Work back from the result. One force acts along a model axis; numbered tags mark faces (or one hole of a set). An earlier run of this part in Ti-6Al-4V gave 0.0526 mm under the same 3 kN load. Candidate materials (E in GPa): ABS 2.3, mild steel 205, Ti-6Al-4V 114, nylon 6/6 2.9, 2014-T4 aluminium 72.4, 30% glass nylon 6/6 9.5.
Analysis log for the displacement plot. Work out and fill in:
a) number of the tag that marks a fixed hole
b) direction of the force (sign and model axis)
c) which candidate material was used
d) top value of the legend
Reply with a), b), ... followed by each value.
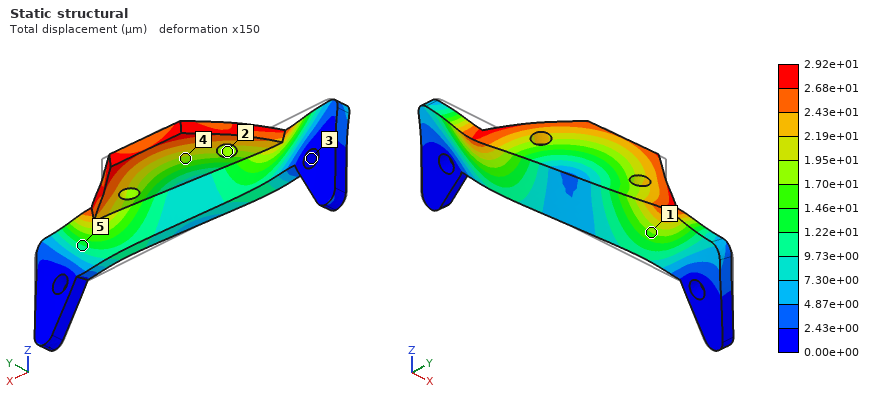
a) 3
b) -X
c) mild steel
d) 2.92e+01 µm
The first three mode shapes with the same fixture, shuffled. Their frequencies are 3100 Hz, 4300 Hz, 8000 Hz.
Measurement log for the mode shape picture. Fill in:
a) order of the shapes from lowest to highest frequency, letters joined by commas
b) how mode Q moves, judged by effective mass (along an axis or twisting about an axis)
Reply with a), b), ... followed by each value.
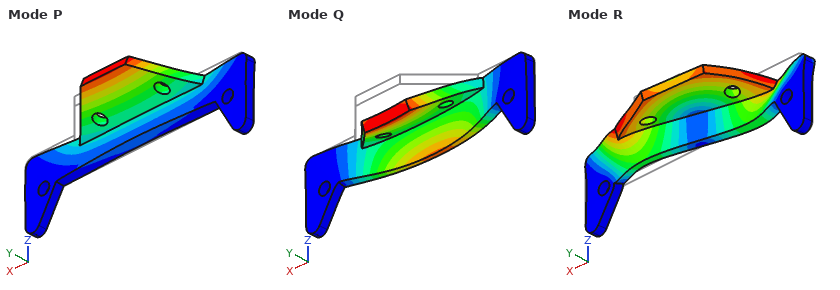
a) P, Q, R
b) along Y
